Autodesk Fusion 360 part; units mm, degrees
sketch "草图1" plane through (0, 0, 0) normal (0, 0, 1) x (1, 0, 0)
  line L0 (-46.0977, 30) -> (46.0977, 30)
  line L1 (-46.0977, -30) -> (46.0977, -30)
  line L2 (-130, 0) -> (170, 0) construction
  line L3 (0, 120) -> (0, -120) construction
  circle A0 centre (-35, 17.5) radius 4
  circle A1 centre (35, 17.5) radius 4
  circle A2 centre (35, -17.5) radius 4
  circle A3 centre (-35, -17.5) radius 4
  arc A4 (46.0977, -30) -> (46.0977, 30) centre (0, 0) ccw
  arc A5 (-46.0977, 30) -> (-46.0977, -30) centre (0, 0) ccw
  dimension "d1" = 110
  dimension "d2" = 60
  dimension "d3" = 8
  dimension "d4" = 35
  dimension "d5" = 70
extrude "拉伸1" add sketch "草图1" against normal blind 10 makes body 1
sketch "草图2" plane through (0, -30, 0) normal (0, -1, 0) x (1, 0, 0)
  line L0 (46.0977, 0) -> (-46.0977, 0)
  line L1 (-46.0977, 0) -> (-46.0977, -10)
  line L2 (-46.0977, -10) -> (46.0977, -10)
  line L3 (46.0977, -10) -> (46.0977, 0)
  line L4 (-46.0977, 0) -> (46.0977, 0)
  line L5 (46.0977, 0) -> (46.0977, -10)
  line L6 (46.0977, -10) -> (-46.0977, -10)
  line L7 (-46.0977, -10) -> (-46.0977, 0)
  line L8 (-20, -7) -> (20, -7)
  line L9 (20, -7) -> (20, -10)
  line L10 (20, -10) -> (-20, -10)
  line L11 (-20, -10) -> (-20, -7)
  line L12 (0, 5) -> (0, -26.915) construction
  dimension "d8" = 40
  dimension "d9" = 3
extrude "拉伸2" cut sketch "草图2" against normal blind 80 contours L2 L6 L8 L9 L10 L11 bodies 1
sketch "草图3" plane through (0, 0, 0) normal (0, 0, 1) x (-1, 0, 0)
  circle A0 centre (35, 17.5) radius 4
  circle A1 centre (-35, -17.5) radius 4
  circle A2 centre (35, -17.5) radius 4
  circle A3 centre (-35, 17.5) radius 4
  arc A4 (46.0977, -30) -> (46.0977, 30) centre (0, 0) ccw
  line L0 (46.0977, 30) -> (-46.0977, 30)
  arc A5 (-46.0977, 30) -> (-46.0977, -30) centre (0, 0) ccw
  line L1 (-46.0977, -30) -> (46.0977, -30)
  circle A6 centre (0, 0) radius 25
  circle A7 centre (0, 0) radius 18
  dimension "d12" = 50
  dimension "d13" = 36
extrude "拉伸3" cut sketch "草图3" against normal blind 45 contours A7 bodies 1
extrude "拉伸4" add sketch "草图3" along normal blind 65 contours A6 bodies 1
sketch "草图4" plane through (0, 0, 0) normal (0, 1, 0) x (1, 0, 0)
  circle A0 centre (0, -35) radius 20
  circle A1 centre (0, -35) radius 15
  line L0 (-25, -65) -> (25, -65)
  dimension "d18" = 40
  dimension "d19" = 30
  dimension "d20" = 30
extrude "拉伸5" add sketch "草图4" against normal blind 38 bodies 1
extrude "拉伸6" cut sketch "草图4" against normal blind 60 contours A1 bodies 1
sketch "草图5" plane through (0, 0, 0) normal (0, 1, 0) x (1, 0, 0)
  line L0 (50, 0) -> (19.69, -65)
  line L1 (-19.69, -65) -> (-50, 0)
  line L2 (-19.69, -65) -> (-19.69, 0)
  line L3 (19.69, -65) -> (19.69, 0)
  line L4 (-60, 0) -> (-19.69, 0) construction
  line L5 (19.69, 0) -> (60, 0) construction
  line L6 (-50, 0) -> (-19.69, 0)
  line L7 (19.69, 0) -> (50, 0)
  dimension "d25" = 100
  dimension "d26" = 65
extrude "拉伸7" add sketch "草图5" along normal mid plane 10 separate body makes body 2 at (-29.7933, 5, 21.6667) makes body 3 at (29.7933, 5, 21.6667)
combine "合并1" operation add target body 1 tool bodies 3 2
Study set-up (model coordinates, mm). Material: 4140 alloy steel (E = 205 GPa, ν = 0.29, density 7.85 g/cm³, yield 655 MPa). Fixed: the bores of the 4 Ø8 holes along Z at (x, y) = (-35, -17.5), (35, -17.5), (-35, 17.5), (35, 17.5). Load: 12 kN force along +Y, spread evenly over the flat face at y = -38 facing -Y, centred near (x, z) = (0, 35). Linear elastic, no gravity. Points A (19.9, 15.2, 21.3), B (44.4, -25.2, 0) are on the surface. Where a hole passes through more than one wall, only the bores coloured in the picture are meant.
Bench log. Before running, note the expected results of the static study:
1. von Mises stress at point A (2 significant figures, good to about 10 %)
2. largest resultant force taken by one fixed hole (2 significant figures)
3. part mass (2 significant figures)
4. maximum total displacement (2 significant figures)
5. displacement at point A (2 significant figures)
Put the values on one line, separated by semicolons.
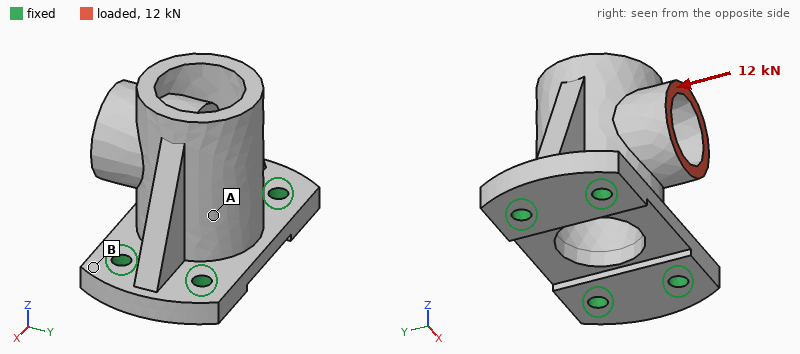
25 MPa; 8.4 kN; 1.0 kg; 99 µm; 35 µm
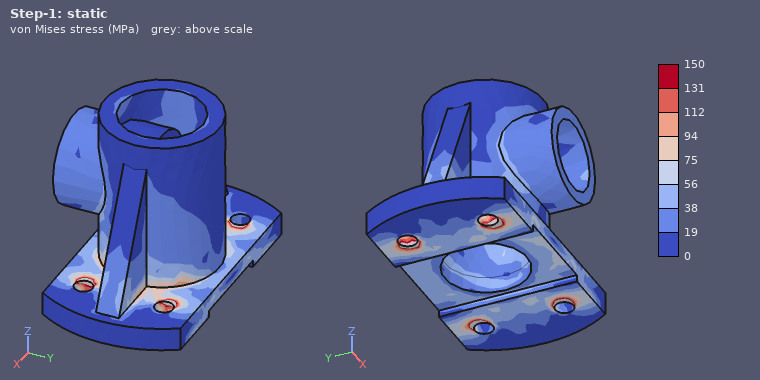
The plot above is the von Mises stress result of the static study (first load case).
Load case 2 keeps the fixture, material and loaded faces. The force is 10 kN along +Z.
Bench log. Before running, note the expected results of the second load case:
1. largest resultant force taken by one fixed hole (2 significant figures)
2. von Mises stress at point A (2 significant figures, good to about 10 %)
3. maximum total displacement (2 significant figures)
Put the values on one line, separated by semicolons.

8.9 kN; 27 MPa; 0.11 mm
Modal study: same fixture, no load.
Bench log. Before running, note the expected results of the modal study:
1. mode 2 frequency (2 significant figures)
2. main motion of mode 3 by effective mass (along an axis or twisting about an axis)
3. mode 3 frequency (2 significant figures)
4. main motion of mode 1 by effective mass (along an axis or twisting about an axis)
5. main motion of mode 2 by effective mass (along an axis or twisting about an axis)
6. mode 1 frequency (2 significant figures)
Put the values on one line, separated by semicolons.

5800 Hz; along Z; 8200 Hz; along Y; along X; 2800 Hz
